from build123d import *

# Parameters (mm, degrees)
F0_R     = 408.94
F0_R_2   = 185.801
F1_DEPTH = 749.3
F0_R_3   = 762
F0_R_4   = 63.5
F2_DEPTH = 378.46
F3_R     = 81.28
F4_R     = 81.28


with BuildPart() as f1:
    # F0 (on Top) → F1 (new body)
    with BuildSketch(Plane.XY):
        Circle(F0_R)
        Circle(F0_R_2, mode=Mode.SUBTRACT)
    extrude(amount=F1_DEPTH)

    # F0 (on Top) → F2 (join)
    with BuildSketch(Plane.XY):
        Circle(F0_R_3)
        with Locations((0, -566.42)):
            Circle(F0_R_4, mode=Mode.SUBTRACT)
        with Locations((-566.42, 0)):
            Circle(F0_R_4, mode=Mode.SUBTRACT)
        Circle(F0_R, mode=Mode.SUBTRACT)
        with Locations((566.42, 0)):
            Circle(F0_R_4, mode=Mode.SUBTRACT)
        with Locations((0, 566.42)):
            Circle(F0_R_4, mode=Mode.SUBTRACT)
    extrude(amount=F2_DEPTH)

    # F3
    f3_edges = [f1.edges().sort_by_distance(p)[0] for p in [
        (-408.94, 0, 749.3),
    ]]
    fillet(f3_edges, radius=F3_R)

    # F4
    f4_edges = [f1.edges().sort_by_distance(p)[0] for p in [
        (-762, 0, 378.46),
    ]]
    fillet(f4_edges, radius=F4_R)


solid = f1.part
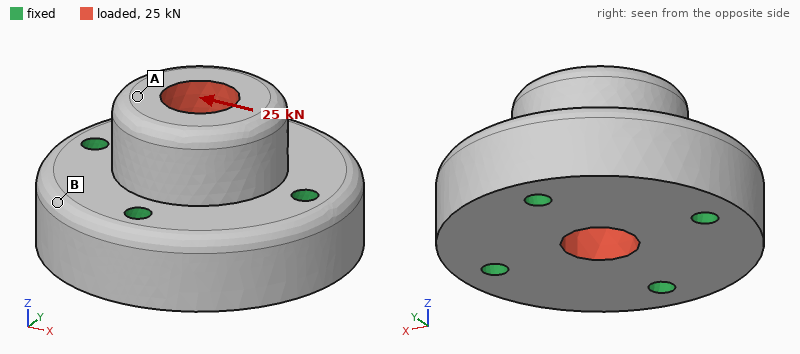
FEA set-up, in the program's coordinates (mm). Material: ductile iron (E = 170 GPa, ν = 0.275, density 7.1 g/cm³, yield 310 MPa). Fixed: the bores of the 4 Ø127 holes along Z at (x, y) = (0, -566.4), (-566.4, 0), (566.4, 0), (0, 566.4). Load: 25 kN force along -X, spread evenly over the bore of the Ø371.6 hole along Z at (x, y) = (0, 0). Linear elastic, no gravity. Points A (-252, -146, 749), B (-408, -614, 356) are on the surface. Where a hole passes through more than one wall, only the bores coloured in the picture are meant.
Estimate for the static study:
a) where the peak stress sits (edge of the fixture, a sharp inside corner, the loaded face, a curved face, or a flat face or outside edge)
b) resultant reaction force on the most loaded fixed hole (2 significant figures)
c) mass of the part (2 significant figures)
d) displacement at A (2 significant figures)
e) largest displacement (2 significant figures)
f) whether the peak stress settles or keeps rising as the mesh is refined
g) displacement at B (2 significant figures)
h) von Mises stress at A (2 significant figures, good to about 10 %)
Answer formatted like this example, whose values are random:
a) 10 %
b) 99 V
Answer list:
a) a sharp inside corner
b) 8.6 kN
c) 5500 kg
d) 0.37 µm
e) 0.40 µm
f) keeps rising
g) 0.068 µm
h) 0.040 MPa
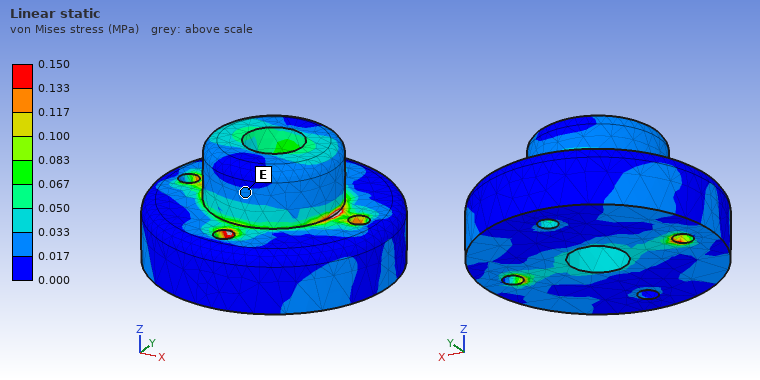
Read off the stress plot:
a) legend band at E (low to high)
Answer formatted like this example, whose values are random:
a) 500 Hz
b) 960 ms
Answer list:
a) 0.017 to 0.033 MPa
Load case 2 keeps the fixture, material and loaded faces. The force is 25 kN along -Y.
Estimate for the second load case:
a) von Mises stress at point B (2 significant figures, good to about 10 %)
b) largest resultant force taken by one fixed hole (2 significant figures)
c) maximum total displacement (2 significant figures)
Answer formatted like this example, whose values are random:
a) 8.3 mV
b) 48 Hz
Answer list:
a) 0.012 MPa
b) 8.6 kN
c) 0.40 µm
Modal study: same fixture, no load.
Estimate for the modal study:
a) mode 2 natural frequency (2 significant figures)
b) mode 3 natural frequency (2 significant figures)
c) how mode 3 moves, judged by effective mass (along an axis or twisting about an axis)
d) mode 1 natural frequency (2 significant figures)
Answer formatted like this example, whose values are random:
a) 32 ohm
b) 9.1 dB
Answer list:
a) 980 Hz
b) 1100 Hz
c) along Z
d) 980 Hz
